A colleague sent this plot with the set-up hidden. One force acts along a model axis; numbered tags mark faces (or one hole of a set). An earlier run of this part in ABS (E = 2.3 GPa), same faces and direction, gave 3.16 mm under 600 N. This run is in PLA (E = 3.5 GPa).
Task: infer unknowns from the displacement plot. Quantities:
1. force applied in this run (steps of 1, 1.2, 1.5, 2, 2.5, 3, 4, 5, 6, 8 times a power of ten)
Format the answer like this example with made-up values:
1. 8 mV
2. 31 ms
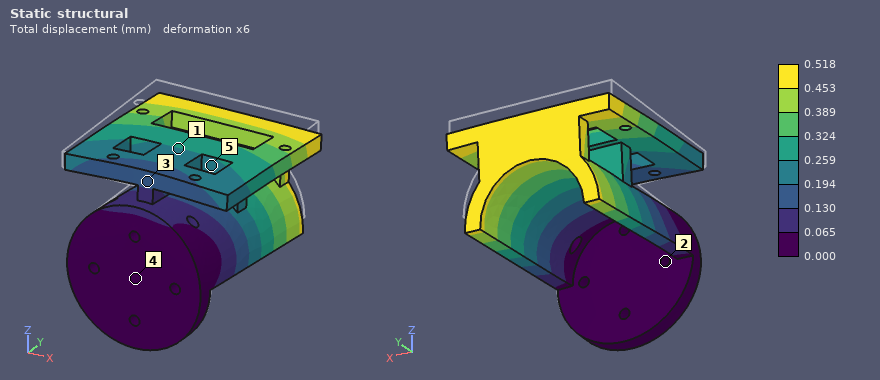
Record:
1. 150 N
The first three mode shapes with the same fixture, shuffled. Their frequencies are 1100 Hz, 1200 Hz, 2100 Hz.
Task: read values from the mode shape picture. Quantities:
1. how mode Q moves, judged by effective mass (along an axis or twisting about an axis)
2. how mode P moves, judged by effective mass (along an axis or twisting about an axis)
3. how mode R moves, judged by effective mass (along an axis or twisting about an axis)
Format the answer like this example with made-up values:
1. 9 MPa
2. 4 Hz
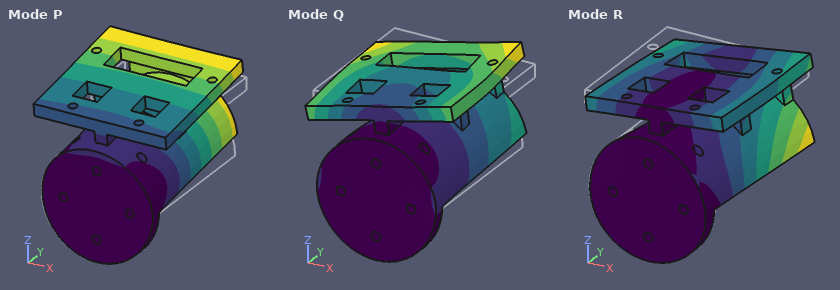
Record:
1. along X
2. along Z
3. along X
